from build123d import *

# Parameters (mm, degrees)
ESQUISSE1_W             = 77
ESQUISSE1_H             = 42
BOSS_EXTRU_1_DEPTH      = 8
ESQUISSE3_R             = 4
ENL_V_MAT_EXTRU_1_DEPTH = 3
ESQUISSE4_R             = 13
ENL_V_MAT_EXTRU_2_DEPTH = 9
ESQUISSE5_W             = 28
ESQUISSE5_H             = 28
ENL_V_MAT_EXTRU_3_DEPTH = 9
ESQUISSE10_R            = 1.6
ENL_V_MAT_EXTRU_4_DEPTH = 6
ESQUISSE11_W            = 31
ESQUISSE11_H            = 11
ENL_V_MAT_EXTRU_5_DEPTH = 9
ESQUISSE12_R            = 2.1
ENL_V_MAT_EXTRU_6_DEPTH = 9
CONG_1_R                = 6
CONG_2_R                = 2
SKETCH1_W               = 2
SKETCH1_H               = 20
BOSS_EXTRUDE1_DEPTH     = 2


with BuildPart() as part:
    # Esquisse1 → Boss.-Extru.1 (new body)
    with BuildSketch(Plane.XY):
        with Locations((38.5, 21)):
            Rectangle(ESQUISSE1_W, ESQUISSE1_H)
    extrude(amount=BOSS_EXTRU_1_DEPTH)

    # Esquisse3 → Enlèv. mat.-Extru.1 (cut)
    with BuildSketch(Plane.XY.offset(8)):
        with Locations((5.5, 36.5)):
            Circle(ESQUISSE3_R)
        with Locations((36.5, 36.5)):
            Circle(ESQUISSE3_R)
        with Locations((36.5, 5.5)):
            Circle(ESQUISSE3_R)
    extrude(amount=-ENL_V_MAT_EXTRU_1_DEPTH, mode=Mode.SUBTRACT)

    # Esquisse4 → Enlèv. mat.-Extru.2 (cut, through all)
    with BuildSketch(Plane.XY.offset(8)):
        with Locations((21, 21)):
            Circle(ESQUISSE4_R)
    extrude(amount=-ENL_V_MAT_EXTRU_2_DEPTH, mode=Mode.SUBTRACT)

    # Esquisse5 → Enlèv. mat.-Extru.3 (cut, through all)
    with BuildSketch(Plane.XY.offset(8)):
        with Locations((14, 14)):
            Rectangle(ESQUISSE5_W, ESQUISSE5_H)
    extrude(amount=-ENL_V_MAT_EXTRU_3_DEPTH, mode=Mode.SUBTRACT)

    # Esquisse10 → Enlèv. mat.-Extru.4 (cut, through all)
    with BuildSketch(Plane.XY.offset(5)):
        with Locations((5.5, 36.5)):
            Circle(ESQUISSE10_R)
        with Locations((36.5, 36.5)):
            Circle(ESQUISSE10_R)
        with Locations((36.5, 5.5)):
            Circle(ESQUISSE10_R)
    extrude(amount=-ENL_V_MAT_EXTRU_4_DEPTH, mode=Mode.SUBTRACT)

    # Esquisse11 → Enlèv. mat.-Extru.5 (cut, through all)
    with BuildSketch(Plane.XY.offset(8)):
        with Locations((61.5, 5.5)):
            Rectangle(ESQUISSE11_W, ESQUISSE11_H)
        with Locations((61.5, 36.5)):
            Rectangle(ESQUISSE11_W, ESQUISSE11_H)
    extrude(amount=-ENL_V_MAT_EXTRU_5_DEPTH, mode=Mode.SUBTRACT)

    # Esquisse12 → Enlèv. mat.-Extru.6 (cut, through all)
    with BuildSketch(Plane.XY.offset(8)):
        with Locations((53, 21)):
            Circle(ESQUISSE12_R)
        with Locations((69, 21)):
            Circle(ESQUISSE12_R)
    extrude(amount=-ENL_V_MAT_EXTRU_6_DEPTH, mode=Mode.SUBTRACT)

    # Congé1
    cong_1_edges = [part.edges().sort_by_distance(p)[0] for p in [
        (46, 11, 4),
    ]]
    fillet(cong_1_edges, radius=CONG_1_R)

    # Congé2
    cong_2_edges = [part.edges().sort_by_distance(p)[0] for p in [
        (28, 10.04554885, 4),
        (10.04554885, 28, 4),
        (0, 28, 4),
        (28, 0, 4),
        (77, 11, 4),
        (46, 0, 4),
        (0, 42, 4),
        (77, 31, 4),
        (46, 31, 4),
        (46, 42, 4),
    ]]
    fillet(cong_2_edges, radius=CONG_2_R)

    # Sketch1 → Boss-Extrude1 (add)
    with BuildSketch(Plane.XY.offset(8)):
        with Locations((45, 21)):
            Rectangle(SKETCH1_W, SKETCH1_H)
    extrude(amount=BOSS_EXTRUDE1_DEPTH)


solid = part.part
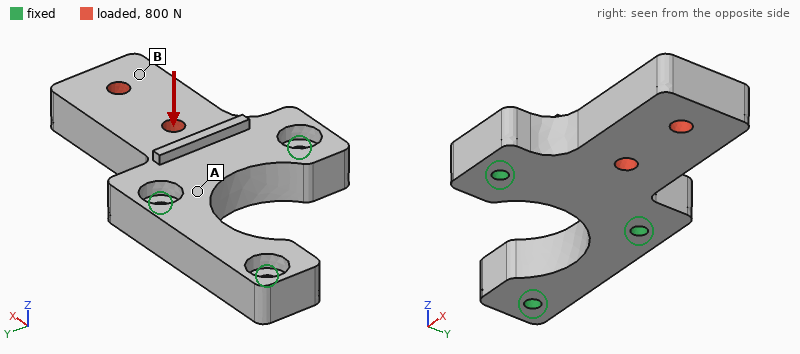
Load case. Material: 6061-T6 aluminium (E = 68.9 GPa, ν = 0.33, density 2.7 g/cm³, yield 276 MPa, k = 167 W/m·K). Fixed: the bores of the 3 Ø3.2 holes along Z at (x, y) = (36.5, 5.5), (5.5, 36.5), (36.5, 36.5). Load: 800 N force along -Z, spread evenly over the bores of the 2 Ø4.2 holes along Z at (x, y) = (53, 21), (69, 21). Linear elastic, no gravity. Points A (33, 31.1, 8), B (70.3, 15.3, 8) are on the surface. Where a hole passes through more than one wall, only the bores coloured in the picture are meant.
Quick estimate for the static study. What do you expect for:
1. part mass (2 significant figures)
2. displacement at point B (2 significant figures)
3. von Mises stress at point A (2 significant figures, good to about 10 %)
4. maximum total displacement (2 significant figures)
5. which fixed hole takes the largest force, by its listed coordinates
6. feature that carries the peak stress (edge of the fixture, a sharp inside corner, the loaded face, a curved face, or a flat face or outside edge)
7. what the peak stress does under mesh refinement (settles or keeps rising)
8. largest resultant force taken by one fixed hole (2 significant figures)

32 g
0.18 mm
58 MPa
0.22 mm
(36.5, 36.5)
edge of the fixture
keeps rising
640 N
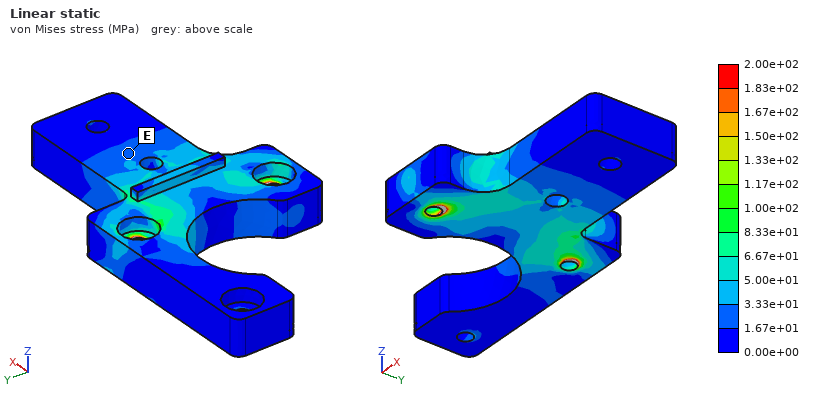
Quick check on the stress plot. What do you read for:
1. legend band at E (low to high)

1.67e+01 to 3.33e+01 MPa
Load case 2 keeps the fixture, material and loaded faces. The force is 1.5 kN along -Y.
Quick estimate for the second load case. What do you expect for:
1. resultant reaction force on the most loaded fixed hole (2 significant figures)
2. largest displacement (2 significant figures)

1.4 kN
36 µm
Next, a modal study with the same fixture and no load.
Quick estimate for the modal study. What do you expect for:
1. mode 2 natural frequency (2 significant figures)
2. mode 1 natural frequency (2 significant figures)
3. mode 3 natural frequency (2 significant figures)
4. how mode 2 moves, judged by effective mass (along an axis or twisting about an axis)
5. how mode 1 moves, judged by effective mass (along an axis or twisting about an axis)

11 kHz
3200 Hz
14 kHz
along Y
along Z
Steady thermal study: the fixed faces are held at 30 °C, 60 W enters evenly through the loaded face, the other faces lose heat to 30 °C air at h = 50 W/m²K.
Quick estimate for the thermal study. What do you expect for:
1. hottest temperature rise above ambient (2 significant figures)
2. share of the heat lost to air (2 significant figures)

60 K
9.0 %
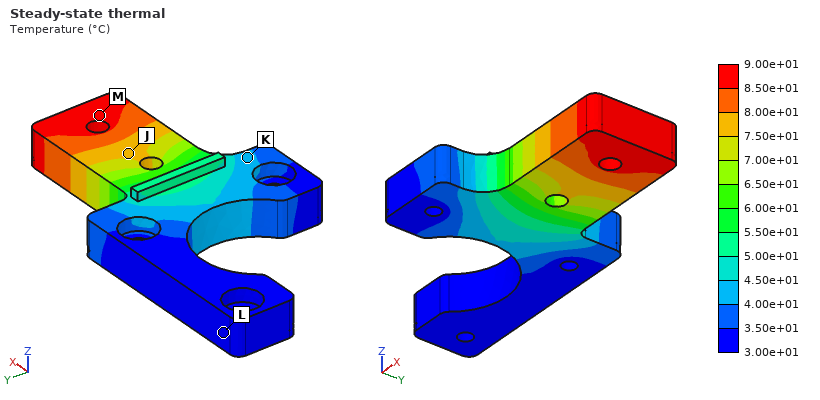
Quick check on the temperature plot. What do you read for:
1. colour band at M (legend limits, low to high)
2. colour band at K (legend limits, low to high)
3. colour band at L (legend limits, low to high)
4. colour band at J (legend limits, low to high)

8.50e+01 to 9.00e+01 °C
4.00e+01 to 4.50e+01 °C
3.00e+01 to 3.50e+01 °C
7.50e+01 to 8.00e+01 °C
